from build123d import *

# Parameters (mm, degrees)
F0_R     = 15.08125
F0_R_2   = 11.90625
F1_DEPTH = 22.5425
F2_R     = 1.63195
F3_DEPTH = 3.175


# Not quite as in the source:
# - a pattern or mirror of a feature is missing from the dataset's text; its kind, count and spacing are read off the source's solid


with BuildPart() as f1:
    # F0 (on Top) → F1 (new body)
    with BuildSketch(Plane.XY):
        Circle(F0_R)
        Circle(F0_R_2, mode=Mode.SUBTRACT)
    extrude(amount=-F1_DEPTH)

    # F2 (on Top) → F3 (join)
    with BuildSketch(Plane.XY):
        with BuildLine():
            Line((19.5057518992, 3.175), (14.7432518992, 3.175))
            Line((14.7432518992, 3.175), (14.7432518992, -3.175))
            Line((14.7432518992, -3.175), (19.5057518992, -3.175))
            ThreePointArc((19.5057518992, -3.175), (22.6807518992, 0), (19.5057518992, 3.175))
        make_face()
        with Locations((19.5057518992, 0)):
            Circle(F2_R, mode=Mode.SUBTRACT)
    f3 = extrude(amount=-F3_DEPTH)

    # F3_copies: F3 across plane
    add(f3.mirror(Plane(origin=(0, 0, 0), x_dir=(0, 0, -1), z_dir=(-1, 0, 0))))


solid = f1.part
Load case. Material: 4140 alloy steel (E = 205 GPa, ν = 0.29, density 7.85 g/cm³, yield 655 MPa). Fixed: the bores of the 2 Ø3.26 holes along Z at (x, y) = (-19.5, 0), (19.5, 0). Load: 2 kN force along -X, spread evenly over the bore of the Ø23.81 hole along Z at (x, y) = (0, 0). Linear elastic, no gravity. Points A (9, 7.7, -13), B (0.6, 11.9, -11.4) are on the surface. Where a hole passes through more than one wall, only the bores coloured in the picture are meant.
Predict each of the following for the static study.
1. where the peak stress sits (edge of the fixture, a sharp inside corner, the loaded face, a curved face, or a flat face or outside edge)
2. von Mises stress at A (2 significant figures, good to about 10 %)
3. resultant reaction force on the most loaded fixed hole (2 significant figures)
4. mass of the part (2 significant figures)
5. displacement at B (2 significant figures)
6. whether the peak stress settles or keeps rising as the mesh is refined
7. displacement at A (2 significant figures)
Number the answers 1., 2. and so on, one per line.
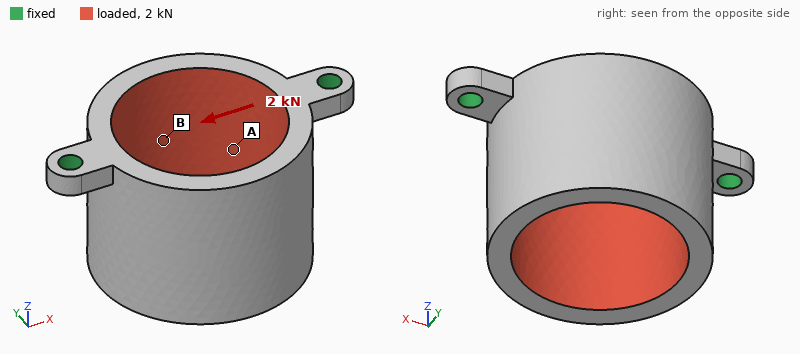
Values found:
1. edge of the fixture
2. 22 MPa
3. 1.2 kN
4. 49 g
5. 8.7 µm
6. keeps rising
7. 8.6 µm
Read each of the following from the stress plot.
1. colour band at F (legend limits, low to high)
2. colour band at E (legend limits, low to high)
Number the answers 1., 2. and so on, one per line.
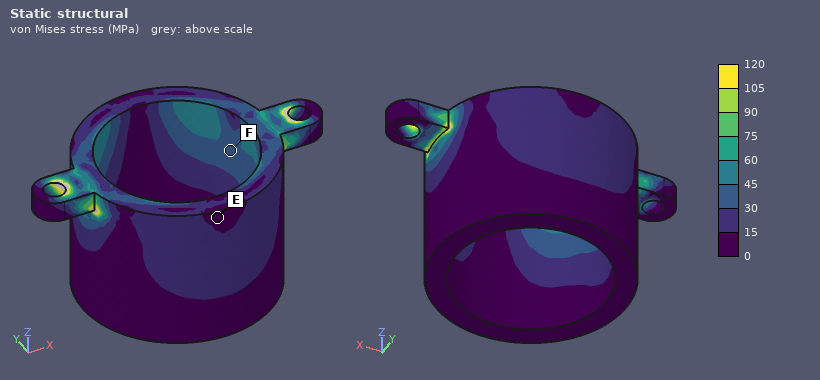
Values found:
1. 30 to 45 MPa
2. 0 to 15 MPa
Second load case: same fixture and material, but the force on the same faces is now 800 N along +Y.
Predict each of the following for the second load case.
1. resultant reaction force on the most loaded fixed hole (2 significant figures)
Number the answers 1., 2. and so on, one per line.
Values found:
1. 400 N
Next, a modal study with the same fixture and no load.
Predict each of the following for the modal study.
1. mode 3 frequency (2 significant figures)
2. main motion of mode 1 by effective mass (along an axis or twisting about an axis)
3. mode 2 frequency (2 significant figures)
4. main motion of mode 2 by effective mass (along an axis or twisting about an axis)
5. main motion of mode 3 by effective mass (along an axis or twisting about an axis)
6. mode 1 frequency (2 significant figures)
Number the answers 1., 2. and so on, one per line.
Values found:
1. 11 kHz
2. along Y
3. 9200 Hz
4. along Z
5. along X
6. 2100 Hz
